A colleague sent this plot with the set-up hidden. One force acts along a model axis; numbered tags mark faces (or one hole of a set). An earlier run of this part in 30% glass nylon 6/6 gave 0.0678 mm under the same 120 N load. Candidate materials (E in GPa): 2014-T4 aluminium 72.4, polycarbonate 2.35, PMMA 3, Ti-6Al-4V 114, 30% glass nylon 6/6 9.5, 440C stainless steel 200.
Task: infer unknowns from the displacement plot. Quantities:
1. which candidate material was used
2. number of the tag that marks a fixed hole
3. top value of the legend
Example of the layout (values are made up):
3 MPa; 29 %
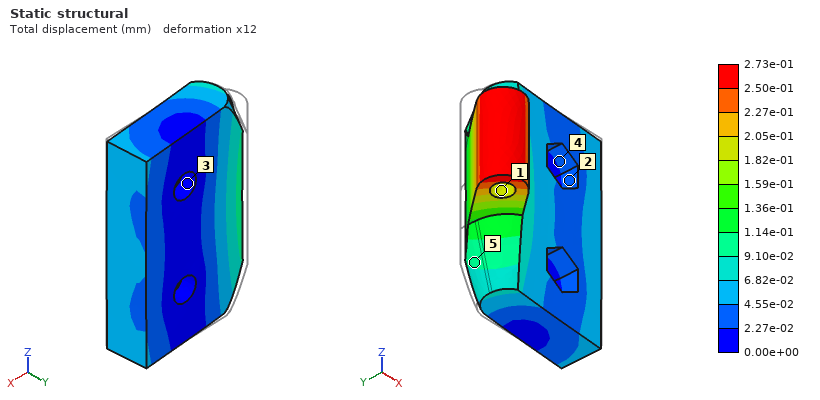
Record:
polycarbonate; 3; 2.73e-01 mm
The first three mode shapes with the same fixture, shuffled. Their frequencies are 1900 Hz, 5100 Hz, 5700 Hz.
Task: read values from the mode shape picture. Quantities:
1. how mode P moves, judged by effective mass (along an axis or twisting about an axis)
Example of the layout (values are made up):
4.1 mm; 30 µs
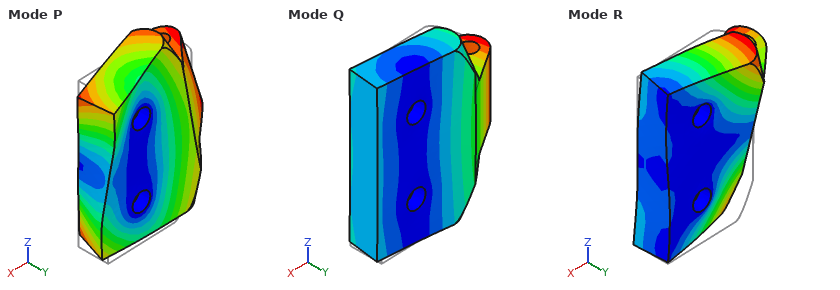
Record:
along Z
